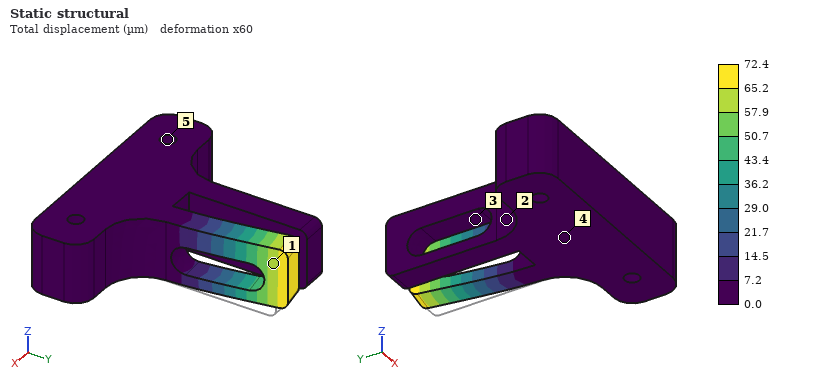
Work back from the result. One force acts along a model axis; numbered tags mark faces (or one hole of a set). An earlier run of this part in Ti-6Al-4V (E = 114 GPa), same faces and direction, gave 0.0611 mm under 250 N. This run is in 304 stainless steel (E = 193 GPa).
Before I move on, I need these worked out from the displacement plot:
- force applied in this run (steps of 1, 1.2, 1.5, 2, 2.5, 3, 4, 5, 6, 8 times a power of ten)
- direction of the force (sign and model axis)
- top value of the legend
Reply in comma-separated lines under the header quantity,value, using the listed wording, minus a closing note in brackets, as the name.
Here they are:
quantity,value
force applied in this run,500 N
direction of the force,-X
top value of the legend,72.4 µm
